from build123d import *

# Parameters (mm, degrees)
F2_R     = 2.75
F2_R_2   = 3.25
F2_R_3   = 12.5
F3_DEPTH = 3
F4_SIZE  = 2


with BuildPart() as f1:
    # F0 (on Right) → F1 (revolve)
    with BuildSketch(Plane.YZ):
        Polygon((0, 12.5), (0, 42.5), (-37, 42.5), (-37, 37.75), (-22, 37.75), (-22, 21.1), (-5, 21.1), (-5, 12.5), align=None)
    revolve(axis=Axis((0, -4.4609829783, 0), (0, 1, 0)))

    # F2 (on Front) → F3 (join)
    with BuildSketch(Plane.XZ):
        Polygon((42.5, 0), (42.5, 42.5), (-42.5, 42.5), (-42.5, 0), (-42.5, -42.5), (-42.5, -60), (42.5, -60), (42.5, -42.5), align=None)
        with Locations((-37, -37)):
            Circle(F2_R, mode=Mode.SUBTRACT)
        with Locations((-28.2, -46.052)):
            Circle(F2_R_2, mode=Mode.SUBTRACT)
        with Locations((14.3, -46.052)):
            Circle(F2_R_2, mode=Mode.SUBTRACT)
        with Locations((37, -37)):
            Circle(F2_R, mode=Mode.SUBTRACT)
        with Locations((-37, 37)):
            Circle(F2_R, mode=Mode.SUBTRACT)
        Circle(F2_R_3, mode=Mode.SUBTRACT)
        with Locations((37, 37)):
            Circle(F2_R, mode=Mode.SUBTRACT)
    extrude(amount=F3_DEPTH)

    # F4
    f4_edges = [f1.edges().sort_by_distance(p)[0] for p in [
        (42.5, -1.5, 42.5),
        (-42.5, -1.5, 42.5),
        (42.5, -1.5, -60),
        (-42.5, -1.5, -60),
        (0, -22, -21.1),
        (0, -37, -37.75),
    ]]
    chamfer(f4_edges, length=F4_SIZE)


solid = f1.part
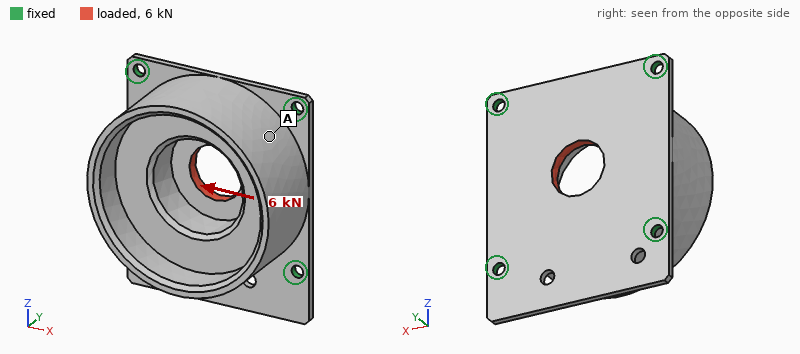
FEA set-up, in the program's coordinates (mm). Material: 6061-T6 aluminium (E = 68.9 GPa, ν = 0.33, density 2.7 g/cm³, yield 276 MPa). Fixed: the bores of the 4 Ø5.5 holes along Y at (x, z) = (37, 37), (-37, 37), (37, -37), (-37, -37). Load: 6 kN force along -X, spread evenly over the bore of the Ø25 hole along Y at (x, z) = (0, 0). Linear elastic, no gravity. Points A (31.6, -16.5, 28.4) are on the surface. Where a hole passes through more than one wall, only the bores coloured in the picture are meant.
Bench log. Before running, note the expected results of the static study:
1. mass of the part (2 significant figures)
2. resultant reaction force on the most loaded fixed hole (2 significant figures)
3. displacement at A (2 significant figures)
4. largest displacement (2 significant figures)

340 g
1.6 kN
8.0 µm
14 µm
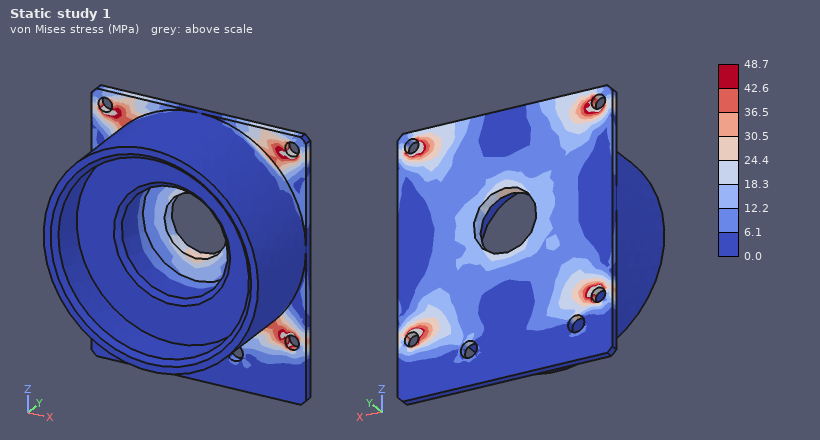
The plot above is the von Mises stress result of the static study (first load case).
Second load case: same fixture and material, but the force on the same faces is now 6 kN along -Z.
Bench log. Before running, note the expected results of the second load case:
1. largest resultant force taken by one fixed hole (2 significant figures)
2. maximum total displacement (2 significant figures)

1.6 kN
14 µm
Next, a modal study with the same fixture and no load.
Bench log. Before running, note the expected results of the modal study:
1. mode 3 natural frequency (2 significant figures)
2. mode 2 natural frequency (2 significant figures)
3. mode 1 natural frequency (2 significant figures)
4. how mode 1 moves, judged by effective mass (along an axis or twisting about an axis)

3400 Hz
3300 Hz
2900 Hz
along Y
